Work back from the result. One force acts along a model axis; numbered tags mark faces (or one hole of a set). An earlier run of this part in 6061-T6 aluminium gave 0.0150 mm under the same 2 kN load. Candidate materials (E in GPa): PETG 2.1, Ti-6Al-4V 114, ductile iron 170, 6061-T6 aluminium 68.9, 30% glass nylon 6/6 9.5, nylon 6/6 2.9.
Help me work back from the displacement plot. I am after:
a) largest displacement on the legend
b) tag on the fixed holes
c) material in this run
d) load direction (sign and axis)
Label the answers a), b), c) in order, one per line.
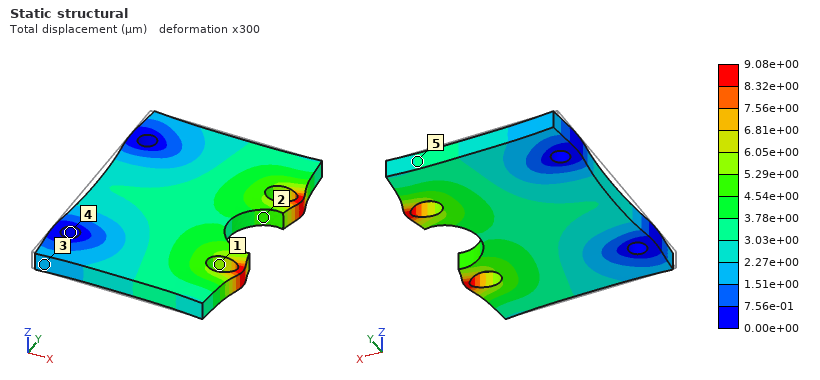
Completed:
a) 9.08e+00 µm
b) 4
c) Ti-6Al-4V
d) +X
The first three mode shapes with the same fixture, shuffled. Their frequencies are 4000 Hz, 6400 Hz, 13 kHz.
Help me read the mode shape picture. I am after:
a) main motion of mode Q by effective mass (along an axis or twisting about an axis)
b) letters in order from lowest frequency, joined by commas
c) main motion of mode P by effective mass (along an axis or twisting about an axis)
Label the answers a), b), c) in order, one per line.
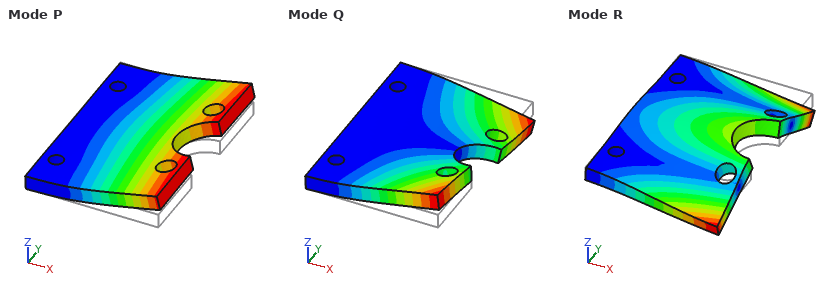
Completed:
a) twisting about X
b) P, Q, R
c) along Z
